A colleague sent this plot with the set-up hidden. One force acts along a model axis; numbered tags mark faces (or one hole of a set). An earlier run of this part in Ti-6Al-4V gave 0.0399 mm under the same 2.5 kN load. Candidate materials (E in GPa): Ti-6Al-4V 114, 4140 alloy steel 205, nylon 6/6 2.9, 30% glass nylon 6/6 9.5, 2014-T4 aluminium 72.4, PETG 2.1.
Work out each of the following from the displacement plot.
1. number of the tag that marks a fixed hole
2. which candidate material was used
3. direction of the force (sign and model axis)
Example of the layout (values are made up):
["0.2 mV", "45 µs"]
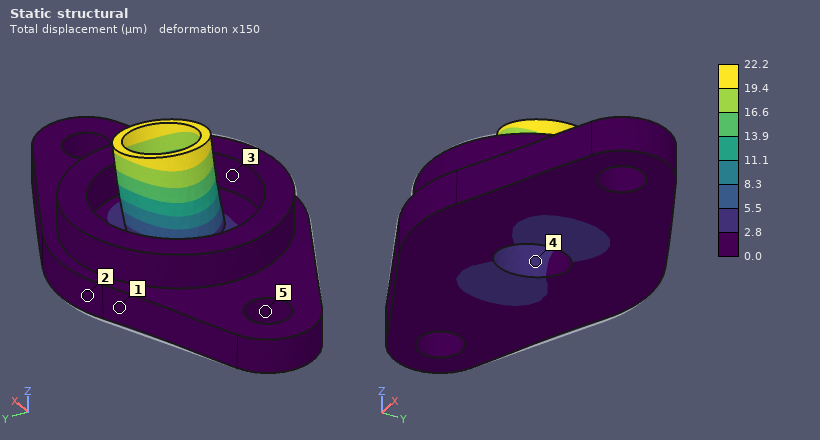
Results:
["5", "4140 alloy steel", "+X"]
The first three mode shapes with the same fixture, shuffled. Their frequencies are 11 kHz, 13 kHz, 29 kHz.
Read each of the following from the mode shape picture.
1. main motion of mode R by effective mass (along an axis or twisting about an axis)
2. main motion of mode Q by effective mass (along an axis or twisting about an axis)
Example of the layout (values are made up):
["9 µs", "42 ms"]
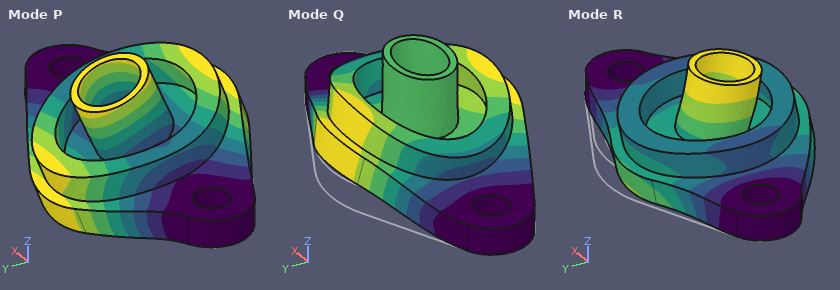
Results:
["along Y", "along Z"]
